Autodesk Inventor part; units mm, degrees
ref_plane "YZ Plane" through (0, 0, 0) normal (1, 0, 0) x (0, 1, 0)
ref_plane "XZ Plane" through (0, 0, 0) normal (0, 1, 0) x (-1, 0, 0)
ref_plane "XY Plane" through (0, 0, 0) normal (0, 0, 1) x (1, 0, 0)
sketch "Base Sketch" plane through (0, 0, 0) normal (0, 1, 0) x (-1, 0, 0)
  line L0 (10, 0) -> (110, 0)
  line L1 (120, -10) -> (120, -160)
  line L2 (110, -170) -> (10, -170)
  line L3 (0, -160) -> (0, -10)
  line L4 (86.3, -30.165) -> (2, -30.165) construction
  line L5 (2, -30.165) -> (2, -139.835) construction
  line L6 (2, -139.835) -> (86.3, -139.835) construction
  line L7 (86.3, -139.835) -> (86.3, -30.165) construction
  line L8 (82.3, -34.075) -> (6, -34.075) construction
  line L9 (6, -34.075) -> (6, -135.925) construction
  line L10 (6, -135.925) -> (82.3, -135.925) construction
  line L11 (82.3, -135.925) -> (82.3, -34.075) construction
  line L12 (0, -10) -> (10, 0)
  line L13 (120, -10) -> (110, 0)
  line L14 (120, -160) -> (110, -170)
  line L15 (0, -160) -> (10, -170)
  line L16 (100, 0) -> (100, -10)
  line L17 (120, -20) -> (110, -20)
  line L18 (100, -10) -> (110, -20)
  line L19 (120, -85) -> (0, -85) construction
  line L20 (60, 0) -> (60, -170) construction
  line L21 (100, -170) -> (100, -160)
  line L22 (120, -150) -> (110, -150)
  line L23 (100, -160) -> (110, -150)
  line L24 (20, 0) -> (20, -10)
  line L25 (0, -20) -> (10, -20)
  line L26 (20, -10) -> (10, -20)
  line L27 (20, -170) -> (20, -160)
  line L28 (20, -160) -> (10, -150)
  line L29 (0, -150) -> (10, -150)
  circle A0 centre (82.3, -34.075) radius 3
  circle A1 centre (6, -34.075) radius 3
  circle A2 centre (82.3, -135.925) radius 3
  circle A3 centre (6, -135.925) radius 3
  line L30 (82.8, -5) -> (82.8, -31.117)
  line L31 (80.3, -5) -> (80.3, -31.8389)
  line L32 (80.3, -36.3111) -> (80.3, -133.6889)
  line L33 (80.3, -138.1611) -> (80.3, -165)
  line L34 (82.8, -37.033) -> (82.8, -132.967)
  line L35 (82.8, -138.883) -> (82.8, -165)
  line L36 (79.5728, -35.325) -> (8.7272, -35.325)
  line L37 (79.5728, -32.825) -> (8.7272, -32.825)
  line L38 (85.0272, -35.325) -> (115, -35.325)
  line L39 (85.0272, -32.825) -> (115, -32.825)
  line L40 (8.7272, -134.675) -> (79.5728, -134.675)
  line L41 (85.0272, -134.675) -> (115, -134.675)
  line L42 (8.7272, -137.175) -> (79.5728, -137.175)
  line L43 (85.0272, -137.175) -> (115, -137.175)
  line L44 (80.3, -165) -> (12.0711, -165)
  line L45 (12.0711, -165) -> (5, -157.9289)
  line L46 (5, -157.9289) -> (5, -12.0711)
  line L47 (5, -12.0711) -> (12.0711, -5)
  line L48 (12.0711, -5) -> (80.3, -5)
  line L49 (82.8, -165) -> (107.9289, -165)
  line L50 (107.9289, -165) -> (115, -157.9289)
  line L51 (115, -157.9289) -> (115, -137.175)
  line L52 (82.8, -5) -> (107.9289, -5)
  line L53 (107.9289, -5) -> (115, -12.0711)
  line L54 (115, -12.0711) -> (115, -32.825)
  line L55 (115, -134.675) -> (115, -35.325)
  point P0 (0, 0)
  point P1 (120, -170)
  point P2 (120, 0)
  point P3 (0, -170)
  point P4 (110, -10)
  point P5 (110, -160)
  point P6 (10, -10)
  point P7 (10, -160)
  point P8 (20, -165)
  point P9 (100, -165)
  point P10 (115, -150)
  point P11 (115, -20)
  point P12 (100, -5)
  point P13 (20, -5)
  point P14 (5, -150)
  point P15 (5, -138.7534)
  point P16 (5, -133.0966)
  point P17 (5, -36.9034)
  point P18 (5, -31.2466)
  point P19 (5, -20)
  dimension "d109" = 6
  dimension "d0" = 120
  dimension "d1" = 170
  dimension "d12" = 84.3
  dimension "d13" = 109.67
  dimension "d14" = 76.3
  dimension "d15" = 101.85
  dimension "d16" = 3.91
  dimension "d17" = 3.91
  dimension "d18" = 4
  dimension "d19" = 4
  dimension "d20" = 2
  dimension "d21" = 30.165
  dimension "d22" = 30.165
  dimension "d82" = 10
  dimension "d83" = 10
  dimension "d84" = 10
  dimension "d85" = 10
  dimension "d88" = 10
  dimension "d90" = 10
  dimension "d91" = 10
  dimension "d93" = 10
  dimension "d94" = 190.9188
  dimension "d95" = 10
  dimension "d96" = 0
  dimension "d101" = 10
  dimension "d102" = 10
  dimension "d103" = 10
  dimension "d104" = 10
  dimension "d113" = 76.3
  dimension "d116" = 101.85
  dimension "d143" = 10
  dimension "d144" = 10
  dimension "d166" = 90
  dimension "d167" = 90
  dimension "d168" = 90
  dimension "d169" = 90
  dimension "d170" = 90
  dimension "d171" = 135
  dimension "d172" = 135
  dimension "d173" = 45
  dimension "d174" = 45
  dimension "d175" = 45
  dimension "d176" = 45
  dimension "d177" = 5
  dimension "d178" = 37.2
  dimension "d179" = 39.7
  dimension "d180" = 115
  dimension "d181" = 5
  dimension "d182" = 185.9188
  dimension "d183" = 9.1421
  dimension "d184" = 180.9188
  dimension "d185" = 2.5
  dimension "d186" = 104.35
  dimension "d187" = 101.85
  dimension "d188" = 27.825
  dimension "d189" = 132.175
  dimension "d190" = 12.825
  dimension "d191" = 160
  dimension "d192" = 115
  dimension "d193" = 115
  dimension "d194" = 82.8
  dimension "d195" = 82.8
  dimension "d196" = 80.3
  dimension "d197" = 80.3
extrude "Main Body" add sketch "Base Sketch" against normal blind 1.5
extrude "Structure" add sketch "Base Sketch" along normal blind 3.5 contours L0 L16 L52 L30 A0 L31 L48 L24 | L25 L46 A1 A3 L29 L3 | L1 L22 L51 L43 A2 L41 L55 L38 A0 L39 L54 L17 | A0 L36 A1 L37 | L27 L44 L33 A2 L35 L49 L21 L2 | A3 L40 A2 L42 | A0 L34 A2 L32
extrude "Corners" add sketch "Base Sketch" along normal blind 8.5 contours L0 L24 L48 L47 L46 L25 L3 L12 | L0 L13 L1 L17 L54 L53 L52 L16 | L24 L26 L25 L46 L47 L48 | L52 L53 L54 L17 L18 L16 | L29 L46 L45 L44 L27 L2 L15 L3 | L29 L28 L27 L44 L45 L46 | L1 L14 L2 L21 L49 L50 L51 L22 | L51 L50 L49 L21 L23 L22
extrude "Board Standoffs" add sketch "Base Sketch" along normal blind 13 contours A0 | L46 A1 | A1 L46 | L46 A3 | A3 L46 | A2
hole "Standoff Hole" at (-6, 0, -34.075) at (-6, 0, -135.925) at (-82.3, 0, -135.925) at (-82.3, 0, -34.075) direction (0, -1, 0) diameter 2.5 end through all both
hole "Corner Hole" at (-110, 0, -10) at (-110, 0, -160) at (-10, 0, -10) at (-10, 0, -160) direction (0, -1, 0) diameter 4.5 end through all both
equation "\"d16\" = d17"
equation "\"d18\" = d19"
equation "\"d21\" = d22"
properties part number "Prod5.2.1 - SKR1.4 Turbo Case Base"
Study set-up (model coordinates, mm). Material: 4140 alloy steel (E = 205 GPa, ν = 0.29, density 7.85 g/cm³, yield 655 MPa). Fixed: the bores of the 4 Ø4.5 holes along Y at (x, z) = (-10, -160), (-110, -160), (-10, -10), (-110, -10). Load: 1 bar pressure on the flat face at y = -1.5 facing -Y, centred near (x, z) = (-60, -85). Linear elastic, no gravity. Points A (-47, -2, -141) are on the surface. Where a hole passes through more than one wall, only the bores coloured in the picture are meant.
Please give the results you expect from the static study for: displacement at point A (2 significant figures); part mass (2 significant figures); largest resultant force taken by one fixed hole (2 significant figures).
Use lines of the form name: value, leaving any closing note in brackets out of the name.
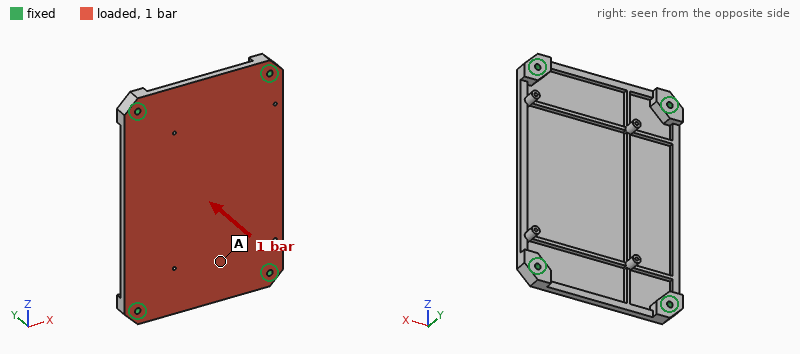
displacement at point A: 0.21 mm
part mass: 400 g
largest resultant force taken by one fixed hole: 620 N
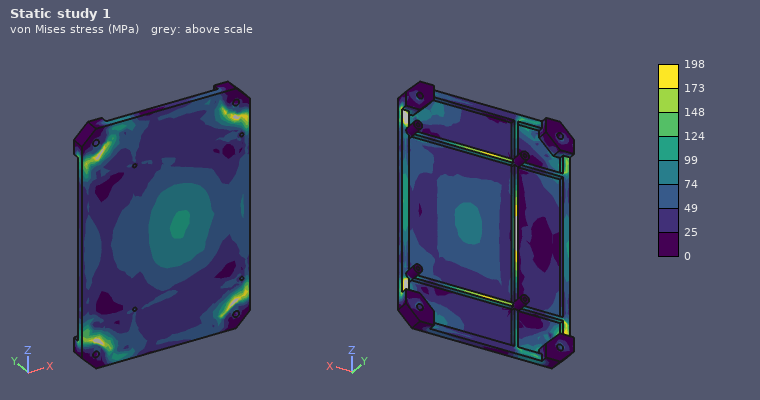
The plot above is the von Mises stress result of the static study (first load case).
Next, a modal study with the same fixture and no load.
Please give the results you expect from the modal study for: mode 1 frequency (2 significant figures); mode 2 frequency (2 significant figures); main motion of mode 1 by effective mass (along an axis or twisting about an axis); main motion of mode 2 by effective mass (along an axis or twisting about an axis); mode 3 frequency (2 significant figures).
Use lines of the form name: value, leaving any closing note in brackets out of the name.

mode 1 frequency: 700 Hz
mode 2 frequency: 1200 Hz
main motion of mode 1 by effective mass: along Y
main motion of mode 2 by effective mass: twisting about Z
mode 3 frequency: 1400 Hz
